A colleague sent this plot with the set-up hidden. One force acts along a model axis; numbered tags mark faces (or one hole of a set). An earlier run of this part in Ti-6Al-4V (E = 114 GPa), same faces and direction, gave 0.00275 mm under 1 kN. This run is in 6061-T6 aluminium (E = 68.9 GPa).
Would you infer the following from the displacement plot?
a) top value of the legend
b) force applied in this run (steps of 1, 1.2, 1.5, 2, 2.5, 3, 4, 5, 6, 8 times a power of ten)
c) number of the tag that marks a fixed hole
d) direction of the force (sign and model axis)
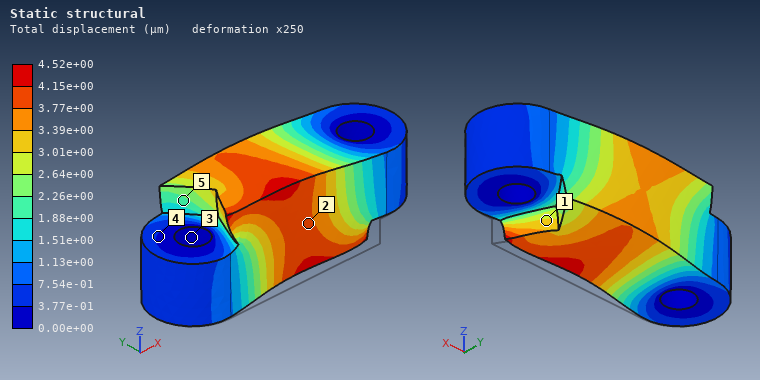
4.52e+00 µm
1 kN
3
+Y
